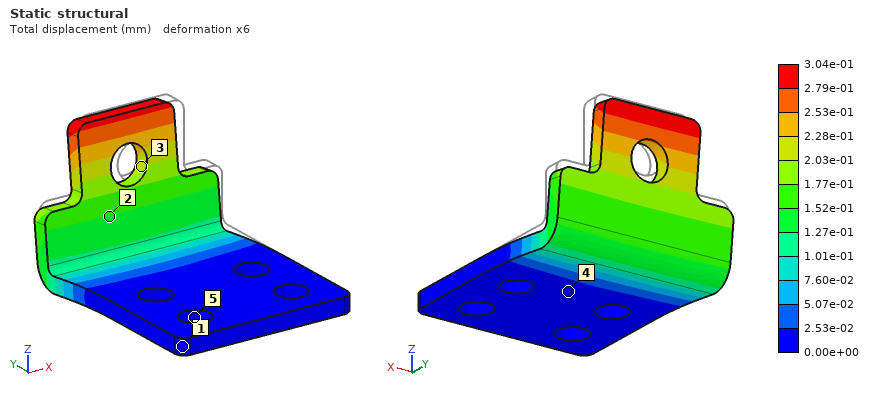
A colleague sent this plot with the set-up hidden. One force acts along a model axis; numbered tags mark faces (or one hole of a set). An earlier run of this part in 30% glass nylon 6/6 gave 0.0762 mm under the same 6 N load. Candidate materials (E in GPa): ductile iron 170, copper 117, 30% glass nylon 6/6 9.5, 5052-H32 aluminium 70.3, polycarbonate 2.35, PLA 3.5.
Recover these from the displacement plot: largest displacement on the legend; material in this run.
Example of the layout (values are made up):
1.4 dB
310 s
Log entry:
3.04e-01 mm
polycarbonate
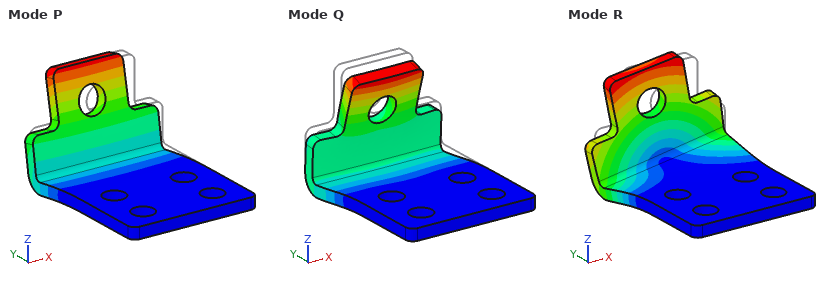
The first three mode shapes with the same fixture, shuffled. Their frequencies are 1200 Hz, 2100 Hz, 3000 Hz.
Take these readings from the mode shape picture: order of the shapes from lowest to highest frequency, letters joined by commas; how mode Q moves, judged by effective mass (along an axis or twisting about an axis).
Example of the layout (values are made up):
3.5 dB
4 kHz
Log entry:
P, R, Q
along Z
